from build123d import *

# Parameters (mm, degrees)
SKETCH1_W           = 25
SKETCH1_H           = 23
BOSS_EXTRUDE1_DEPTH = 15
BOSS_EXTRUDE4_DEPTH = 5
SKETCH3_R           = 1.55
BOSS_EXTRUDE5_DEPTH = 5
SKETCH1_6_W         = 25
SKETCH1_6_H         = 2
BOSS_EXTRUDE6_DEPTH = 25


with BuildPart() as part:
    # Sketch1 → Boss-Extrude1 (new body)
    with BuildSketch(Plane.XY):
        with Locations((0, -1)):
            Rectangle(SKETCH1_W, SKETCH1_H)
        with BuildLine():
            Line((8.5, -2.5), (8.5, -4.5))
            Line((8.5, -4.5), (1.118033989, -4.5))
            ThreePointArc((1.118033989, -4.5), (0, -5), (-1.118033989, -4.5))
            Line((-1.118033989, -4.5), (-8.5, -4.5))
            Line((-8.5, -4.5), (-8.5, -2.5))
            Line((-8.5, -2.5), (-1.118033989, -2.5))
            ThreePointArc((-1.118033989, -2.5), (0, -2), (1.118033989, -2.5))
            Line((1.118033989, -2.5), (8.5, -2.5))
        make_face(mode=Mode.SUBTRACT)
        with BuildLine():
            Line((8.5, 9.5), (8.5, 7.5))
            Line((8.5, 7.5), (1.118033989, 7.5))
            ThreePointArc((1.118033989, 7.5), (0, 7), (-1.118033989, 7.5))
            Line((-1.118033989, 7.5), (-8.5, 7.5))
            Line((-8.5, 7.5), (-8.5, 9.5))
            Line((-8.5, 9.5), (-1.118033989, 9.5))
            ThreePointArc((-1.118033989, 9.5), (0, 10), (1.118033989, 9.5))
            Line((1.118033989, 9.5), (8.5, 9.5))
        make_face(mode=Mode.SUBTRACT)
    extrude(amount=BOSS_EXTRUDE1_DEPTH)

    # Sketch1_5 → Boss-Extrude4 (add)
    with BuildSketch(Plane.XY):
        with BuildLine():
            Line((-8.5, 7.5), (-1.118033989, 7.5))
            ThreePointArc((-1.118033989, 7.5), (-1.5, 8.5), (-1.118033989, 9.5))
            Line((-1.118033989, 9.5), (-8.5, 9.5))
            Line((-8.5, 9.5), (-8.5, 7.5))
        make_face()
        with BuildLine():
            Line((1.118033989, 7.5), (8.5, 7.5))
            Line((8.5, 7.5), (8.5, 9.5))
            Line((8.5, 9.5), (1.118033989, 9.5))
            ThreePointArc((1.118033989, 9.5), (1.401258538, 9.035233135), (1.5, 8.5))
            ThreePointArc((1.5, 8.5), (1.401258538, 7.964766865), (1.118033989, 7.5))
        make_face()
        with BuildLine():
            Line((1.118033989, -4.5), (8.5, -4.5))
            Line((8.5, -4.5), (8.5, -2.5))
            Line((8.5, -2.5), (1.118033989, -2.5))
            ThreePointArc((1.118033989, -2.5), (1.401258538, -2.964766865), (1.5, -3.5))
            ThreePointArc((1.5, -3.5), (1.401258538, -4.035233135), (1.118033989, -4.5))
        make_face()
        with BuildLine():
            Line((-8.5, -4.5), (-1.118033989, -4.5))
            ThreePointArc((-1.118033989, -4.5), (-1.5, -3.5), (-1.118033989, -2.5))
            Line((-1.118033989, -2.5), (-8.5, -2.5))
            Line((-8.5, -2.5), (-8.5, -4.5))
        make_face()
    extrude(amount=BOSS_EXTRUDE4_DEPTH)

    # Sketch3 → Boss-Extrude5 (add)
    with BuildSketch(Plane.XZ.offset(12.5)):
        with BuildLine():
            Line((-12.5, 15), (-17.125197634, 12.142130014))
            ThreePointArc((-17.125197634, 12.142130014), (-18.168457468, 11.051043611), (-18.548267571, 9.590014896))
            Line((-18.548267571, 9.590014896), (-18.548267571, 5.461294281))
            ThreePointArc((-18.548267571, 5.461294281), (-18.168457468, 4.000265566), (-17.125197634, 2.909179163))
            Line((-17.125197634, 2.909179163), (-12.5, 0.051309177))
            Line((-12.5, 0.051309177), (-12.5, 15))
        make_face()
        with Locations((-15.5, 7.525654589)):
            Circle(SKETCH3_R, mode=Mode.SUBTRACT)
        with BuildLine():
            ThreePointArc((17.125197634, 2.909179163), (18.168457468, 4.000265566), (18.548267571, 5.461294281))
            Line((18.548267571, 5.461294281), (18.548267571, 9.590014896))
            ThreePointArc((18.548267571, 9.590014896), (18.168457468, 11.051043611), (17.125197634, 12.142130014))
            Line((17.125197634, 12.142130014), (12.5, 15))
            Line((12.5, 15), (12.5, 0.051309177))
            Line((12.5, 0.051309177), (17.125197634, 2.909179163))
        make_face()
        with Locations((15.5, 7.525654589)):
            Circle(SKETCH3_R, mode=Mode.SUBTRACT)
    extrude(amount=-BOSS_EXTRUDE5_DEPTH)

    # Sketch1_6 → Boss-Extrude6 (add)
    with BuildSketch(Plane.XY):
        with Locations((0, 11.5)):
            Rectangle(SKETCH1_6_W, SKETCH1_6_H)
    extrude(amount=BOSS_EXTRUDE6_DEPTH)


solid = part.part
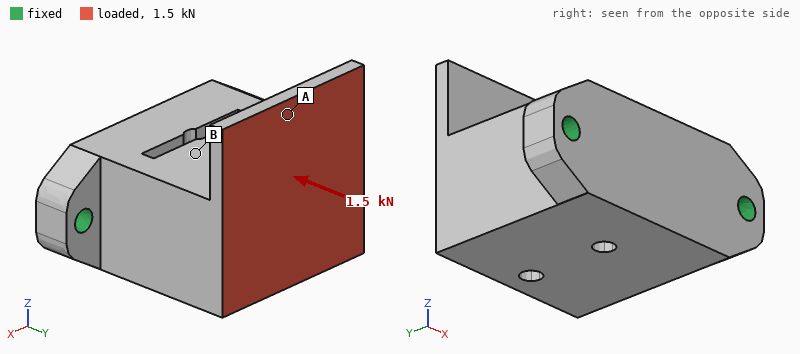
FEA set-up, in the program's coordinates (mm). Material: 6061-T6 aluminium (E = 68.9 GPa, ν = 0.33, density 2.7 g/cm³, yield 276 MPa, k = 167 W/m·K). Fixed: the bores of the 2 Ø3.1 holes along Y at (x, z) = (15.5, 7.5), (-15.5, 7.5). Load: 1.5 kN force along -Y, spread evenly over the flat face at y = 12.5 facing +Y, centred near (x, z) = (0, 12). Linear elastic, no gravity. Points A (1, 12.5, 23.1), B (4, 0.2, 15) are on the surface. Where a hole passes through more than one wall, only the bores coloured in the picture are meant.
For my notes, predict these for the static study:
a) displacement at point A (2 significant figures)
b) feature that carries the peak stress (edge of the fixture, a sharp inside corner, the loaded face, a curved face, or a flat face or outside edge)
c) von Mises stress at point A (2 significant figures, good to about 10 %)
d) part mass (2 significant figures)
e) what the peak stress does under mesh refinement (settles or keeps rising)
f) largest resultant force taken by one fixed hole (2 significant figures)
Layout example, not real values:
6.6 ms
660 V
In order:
0.17 mm
a sharp inside corner
40 MPa
26 g
keeps rising
780 N
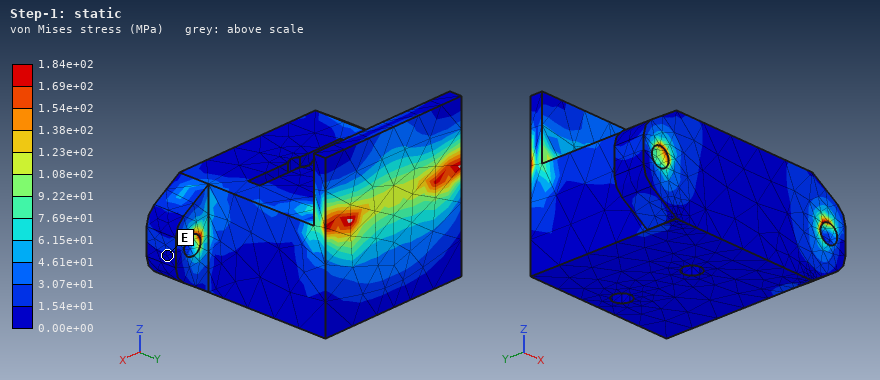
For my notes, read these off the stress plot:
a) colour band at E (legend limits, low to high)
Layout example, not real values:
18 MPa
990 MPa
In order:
0.00e+00 to 1.54e+01 MPa
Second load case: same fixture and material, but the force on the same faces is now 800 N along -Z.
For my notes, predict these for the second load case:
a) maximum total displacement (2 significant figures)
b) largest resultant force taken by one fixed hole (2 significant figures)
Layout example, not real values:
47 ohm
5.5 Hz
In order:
0.13 mm
400 N
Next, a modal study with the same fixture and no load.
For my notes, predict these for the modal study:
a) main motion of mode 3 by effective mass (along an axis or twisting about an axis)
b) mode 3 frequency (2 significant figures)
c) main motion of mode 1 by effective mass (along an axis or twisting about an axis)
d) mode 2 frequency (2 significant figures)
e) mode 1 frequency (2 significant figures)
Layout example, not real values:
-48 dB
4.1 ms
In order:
along X
13 kHz
along Z
11 kHz
4900 Hz
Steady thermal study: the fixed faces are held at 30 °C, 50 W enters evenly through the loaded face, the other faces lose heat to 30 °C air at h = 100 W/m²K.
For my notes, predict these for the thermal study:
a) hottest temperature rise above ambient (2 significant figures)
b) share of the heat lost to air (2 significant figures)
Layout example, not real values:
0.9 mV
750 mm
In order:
56 K
16 %
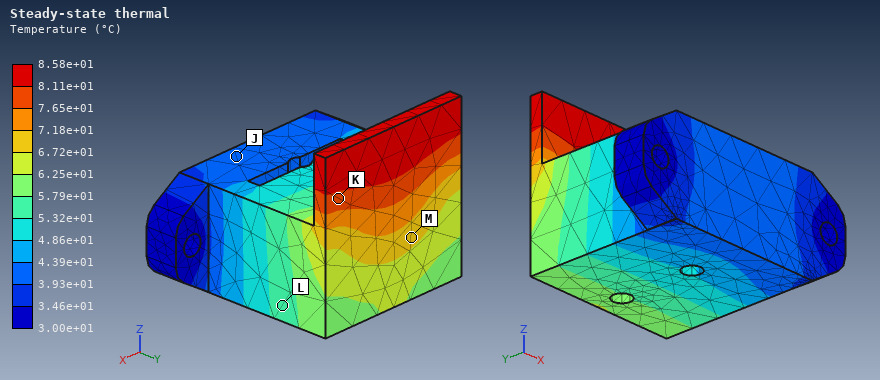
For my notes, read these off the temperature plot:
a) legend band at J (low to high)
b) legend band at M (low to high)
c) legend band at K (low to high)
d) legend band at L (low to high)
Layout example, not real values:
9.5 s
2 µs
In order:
3.93e+01 to 4.39e+01 °C
6.72e+01 to 7.18e+01 °C
7.65e+01 to 8.11e+01 °C
5.32e+01 to 5.79e+01 °C
